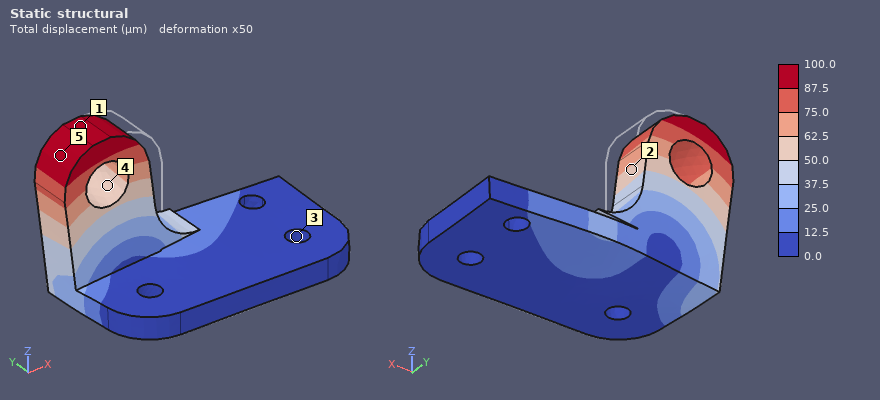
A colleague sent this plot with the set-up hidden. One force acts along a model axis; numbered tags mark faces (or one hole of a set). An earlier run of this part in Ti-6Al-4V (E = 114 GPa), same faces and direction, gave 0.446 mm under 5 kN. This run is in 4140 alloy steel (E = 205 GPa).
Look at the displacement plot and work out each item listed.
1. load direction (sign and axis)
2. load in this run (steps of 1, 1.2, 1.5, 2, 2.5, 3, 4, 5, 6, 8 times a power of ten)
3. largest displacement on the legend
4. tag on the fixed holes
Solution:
-X
2 kN
100.0 µm
3
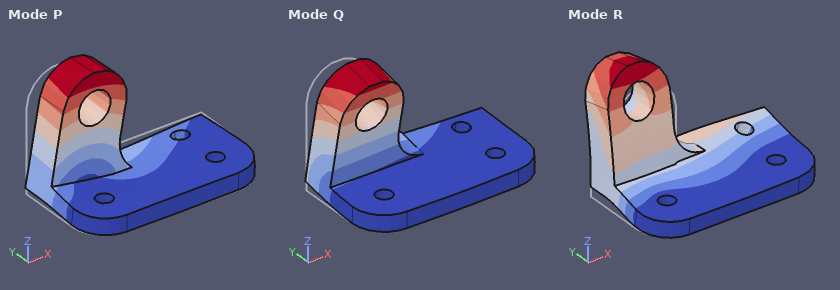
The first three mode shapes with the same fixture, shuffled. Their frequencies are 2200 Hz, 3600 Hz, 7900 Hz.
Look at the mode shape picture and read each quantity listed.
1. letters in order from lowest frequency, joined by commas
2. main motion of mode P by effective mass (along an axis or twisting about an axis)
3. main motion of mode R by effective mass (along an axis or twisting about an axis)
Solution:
Q, P, R
along X
along Z
